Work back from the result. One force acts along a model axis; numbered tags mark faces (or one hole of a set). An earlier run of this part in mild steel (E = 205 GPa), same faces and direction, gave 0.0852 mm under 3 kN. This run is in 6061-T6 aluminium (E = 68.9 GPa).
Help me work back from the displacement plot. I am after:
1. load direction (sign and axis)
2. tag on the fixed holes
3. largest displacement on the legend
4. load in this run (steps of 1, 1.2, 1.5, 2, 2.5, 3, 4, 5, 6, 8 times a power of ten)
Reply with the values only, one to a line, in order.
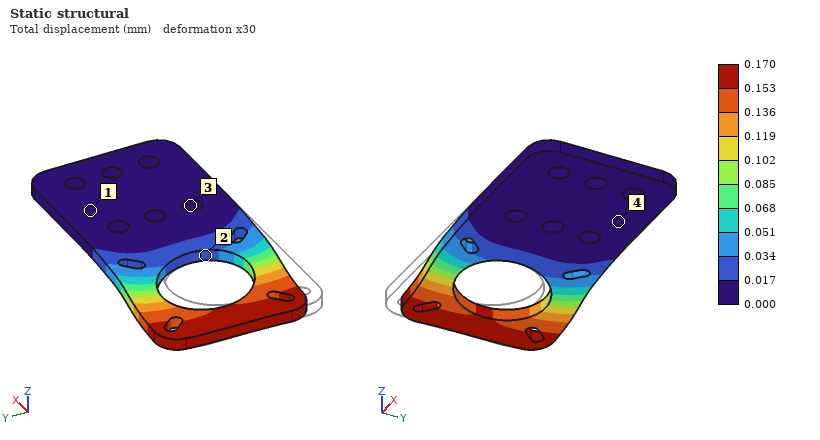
+Y
3
0.170 mm
2 kN
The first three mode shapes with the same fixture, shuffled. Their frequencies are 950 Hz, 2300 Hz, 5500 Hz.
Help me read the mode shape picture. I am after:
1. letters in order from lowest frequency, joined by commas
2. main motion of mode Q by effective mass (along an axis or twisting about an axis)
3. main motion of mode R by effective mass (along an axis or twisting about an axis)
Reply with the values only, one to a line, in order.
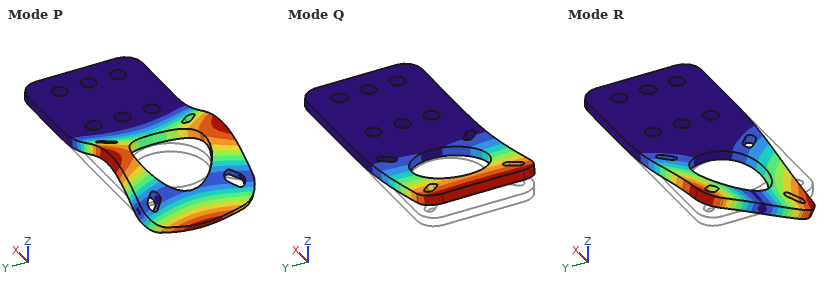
Q, R, P
along Z
twisting about X
